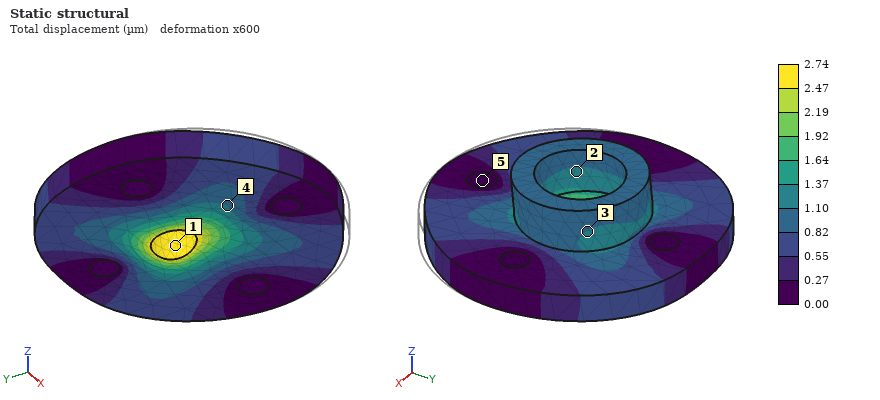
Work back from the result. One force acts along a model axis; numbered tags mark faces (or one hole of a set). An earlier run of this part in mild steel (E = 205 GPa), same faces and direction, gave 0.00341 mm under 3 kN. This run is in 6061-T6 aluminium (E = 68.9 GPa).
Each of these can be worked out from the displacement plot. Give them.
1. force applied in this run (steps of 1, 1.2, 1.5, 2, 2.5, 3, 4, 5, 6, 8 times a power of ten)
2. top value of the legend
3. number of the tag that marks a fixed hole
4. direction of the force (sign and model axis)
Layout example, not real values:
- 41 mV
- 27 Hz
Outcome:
- 800 N
- 2.74 µm
- 5
- +Y
